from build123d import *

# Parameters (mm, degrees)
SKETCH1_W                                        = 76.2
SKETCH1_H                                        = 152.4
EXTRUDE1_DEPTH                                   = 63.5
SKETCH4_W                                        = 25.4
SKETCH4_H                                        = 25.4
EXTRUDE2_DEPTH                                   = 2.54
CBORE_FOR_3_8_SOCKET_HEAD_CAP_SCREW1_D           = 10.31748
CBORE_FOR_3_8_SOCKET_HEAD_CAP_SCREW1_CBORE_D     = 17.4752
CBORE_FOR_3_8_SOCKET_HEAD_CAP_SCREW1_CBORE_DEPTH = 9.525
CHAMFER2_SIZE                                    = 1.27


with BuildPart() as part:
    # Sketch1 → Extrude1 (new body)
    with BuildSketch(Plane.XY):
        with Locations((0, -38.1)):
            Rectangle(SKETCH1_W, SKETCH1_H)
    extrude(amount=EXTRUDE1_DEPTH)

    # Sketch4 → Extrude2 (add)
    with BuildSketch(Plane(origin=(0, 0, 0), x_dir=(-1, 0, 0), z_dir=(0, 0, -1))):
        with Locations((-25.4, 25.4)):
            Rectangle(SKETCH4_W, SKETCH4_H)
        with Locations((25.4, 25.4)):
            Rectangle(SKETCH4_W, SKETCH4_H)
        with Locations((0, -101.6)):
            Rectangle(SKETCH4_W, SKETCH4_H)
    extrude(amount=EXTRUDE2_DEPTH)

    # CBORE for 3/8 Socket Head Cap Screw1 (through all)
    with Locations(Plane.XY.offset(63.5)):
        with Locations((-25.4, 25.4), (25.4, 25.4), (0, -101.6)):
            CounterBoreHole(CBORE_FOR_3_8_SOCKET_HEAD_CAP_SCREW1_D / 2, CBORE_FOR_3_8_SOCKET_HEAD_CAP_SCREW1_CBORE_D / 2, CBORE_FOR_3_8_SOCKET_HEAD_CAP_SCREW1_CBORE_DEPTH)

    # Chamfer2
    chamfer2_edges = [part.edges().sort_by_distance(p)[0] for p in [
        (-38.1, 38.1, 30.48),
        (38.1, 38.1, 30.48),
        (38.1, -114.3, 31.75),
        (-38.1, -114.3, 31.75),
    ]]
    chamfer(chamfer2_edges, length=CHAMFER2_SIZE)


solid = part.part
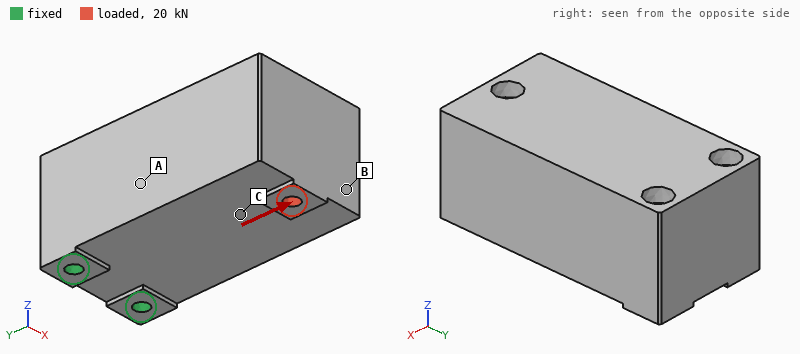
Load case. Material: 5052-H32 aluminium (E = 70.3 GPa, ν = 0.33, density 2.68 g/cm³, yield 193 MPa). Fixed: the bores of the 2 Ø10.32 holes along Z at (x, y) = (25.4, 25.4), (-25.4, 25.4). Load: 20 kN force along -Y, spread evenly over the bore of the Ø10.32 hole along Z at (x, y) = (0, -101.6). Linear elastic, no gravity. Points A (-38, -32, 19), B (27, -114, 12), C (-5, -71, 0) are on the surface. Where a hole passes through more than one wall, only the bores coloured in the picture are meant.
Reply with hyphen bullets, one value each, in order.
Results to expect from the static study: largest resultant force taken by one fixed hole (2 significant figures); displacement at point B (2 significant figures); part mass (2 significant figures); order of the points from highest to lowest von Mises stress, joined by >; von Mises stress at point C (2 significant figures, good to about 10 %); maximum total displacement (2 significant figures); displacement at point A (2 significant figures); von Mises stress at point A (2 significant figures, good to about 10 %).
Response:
- 10 kN
- 12 µm
- 1.9 kg
- C > A > B
- 9.4 MPa
- 19 µm
- 4.7 µm
- 5.1 MPa
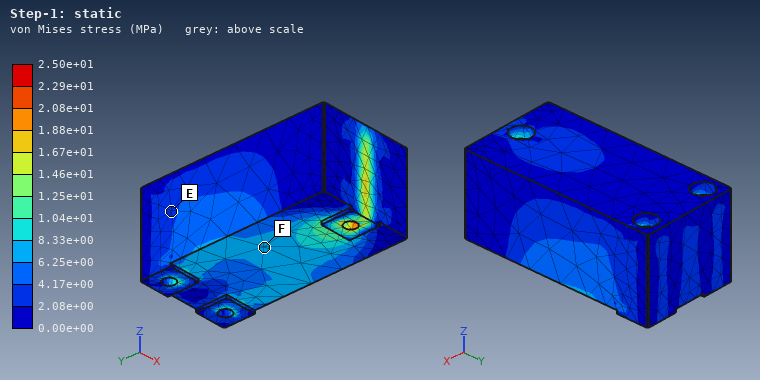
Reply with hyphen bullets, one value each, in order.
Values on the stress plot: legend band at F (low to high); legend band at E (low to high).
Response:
- 6.25e+00 to 8.33e+00 MPa
- 2.08e+00 to 4.17e+00 MPa
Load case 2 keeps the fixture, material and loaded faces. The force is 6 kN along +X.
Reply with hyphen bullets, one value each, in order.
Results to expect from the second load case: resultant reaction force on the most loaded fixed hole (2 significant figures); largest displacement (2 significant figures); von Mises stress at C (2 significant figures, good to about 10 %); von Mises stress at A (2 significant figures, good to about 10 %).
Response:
- 14 kN
- 41 µm
- 4.3 MPa
- 7.1 MPa
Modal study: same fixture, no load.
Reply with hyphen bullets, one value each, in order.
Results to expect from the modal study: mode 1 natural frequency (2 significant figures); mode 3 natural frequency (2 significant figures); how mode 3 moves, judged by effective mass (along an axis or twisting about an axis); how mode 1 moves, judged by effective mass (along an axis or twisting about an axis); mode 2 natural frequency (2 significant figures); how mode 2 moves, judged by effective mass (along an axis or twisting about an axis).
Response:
- 2100 Hz
- 5100 Hz
- twisting about Y
- along Z
- 2700 Hz
- along X
